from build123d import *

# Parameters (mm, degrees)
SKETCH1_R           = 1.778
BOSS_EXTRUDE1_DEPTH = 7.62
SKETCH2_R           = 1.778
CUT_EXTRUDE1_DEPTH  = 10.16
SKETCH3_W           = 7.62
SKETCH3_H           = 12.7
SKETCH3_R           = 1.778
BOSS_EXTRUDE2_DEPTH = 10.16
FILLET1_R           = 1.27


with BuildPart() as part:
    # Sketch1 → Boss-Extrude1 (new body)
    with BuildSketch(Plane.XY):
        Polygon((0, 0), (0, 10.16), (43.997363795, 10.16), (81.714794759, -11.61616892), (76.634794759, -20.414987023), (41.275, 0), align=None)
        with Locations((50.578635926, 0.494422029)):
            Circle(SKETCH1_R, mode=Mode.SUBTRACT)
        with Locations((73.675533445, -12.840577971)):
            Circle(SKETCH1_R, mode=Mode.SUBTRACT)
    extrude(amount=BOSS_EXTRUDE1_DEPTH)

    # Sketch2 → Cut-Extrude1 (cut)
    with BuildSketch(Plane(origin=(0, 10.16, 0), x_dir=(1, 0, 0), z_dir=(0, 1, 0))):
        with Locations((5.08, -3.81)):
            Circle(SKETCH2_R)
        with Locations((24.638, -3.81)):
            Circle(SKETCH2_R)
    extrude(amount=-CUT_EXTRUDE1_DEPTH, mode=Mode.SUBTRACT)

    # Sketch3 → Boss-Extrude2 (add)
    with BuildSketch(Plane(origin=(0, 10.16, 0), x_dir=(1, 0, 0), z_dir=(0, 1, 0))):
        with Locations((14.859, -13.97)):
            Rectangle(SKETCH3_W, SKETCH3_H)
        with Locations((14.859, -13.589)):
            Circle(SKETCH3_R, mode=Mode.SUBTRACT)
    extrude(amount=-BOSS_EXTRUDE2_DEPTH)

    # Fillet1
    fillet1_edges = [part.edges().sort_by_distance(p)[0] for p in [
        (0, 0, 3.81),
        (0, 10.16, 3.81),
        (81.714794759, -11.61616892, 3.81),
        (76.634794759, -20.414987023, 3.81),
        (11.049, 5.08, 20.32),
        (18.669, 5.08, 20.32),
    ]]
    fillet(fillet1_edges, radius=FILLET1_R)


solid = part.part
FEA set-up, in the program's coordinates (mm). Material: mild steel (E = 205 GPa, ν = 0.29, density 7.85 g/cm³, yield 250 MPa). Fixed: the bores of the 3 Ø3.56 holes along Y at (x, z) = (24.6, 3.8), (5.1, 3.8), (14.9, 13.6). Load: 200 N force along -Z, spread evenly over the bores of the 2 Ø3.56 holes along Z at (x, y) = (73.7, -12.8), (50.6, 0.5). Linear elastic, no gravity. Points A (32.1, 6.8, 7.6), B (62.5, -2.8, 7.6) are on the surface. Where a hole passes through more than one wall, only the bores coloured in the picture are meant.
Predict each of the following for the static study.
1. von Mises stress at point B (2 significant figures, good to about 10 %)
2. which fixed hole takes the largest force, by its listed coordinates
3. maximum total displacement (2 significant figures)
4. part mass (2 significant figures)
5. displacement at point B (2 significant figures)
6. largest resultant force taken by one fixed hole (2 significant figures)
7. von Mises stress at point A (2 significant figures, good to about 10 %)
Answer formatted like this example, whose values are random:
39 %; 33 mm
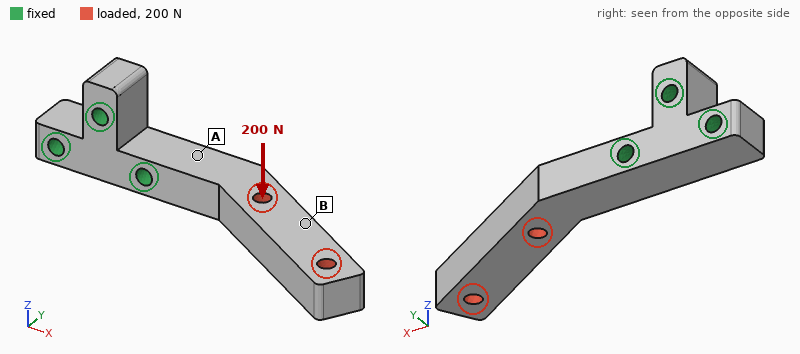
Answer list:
15 MPa; (24.6, 3.8); 0.11 mm; 56 g; 0.059 mm; 350 N; 66 MPa
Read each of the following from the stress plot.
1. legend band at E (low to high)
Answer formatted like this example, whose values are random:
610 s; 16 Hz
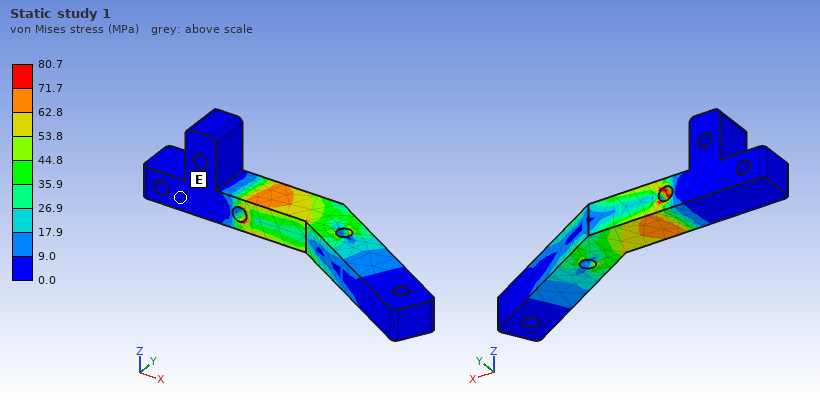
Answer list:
0.0 to 9.0 MPa
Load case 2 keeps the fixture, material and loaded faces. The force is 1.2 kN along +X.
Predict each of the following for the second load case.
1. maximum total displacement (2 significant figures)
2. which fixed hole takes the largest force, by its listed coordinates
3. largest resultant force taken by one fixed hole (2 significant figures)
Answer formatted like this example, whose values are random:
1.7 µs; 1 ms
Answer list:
0.13 mm; (24.6, 3.8); 1.2 kN
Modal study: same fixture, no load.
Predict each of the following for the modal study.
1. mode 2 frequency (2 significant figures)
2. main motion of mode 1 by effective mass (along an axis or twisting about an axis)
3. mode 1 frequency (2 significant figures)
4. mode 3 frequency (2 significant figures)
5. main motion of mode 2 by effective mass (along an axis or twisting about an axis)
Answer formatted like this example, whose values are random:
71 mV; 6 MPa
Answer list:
2400 Hz; along Z; 1700 Hz; 9100 Hz; along Y
